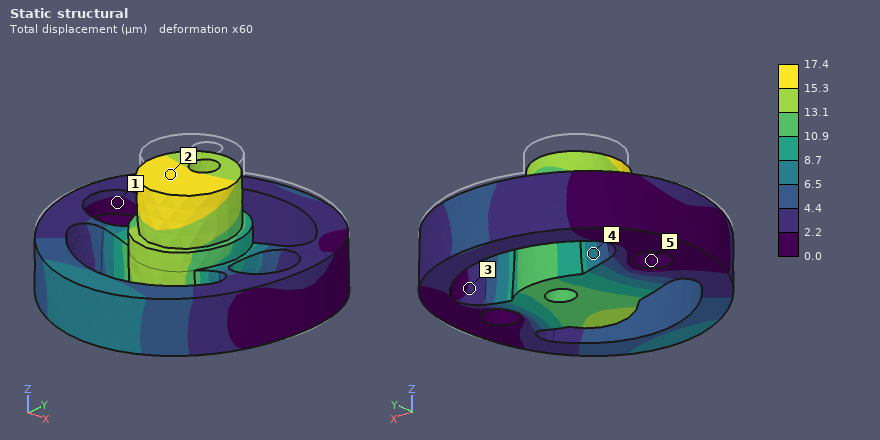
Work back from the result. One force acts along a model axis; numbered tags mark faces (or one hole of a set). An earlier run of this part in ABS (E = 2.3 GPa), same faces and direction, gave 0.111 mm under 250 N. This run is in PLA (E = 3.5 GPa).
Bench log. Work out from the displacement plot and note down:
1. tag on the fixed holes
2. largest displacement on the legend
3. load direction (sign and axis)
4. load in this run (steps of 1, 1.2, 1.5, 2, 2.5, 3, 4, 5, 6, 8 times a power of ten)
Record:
5
17.4 µm
-Z
60 N
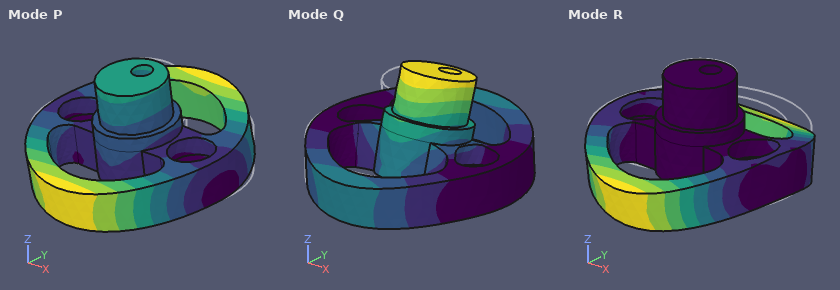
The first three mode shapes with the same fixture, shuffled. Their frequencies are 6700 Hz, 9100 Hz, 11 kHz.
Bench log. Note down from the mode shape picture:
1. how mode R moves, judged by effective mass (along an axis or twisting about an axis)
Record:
along Z
